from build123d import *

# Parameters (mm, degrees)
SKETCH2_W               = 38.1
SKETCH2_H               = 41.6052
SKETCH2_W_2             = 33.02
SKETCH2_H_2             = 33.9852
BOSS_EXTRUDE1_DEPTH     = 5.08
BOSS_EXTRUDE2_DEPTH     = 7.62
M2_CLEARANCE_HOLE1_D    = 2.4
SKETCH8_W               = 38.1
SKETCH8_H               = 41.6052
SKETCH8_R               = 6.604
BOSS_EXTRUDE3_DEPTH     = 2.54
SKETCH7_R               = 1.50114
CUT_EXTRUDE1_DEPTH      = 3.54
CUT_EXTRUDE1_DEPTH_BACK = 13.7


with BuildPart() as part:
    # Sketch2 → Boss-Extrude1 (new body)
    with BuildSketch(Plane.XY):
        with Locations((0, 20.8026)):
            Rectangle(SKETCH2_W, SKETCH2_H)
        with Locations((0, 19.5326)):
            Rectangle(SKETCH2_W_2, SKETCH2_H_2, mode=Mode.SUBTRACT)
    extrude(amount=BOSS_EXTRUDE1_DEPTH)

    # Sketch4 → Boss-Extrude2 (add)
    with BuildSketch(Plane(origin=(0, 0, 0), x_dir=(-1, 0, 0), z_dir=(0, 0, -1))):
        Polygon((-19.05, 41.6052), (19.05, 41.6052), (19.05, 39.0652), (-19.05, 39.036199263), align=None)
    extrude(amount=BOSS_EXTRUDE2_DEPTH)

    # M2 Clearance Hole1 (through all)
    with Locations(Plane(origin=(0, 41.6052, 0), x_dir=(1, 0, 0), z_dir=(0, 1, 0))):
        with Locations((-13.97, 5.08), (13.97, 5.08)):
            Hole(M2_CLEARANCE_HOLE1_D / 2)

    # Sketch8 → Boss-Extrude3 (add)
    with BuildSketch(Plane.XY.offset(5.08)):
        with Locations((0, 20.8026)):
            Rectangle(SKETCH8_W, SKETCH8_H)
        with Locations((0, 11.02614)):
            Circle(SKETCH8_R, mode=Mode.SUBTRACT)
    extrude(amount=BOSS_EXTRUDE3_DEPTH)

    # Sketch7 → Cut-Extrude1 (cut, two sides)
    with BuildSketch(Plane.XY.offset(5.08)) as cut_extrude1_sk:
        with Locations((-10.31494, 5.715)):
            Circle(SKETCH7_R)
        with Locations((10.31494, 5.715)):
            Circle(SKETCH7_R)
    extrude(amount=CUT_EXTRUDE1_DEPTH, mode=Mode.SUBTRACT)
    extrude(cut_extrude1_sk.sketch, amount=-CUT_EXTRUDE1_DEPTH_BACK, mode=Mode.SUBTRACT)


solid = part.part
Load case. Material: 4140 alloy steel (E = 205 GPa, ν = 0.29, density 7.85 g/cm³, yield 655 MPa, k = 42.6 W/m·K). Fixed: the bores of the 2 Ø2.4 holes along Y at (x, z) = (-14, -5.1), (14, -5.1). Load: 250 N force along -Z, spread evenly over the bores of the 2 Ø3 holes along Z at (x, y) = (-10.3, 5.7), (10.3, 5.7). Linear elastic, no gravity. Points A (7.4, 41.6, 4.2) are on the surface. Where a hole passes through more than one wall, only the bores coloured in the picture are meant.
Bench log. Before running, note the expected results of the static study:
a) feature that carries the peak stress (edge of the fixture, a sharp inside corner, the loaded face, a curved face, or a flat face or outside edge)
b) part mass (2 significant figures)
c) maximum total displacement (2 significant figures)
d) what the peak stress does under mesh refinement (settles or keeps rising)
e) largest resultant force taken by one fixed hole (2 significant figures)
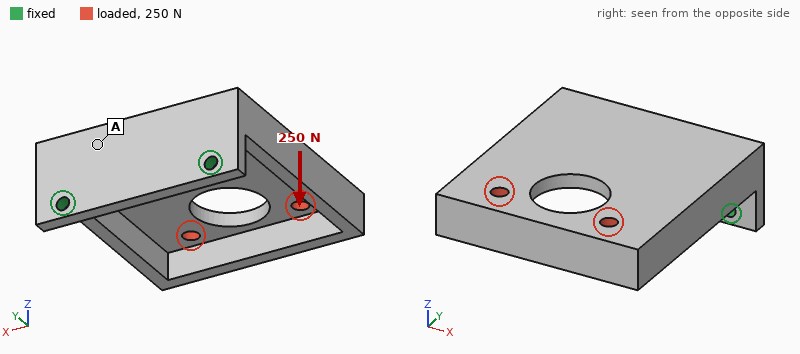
edge of the fixture
53 g
0.37 mm
keeps rising
130 N
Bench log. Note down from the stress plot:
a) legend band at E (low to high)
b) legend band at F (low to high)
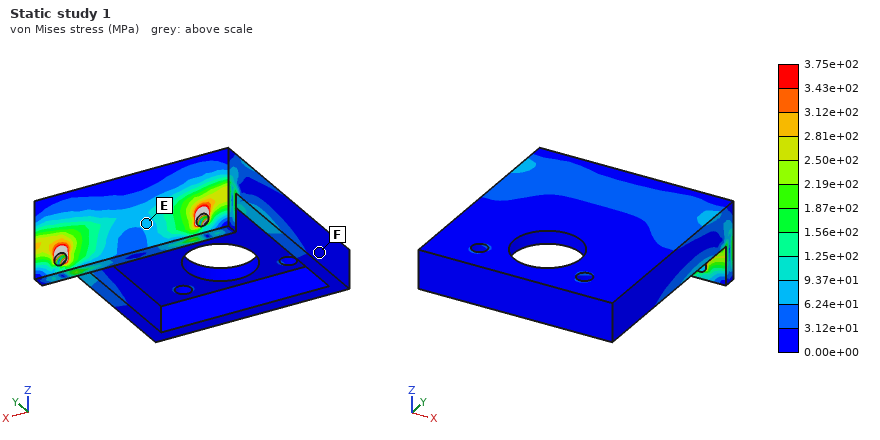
6.24e+01 to 9.37e+01 MPa
0.00e+00 to 3.12e+01 MPa
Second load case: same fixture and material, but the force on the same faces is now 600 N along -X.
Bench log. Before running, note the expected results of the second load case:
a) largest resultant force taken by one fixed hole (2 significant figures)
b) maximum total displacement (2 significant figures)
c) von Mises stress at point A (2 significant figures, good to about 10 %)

790 N
0.11 mm
72 MPa
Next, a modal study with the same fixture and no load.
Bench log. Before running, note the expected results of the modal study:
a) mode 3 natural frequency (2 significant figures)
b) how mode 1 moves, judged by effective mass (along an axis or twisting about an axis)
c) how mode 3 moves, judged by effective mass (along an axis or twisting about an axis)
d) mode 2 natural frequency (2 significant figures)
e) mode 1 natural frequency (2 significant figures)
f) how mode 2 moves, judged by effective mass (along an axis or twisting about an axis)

5200 Hz
along Z
along X
2500 Hz
1000 Hz
along X
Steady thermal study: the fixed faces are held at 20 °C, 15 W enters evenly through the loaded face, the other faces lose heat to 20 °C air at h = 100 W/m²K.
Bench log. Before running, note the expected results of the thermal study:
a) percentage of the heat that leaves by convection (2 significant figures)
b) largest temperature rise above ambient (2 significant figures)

83 %
64 K
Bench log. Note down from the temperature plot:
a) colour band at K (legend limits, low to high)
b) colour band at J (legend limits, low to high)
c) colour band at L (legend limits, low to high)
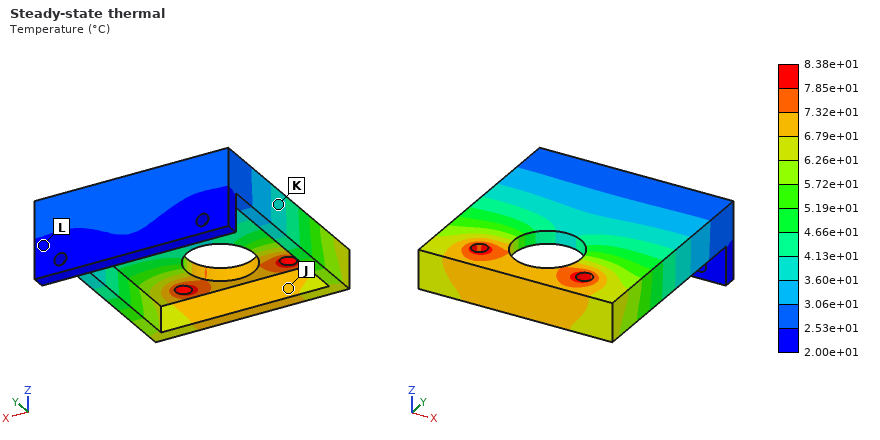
3.60e+01 to 4.13e+01 °C
6.79e+01 to 7.32e+01 °C
2.00e+01 to 2.53e+01 °C
